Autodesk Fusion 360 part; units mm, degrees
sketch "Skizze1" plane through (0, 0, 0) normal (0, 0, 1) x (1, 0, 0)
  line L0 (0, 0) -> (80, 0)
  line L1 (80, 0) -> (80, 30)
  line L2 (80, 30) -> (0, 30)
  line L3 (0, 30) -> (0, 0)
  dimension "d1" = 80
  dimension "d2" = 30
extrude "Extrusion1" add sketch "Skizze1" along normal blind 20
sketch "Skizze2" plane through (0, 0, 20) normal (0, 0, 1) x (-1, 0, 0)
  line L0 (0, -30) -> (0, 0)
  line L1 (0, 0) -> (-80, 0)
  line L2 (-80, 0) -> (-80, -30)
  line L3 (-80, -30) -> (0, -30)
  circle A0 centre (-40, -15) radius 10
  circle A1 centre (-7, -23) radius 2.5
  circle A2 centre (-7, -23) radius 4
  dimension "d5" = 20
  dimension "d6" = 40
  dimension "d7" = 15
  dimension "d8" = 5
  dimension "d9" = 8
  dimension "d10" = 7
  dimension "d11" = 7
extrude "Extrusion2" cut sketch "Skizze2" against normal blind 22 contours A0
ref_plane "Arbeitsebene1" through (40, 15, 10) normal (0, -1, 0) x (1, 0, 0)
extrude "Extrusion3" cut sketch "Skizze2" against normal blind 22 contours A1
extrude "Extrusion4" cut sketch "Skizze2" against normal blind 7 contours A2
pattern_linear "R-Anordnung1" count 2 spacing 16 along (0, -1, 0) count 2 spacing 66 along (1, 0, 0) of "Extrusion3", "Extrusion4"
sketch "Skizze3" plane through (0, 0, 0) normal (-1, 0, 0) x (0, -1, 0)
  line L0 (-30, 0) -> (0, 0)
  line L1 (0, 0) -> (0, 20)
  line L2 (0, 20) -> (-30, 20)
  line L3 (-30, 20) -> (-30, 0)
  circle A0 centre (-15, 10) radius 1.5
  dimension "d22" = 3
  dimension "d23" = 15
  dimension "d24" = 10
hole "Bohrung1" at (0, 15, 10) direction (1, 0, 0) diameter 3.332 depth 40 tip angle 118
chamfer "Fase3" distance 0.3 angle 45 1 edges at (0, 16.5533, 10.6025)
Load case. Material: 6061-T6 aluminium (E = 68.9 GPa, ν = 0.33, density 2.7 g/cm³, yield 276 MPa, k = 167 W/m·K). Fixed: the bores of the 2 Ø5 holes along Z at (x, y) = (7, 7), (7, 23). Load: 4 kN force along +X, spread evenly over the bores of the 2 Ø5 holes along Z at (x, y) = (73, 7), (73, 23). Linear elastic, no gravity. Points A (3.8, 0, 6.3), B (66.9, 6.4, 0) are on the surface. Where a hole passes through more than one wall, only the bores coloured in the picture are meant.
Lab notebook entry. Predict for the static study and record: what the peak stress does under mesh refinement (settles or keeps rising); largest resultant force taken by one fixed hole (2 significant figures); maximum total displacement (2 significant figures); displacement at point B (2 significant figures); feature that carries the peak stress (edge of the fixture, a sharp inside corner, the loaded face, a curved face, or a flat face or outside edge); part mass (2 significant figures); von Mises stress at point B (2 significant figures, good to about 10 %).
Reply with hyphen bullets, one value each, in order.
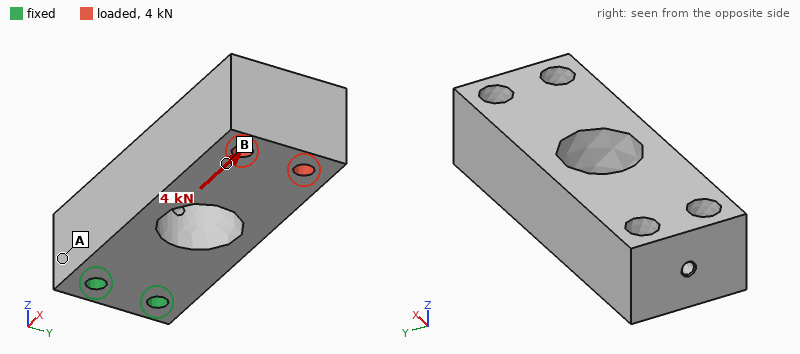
- keeps rising
- 2.0 kN
- 47 µm
- 35 µm
- a sharp inside corner
- 110 g
- 13 MPa
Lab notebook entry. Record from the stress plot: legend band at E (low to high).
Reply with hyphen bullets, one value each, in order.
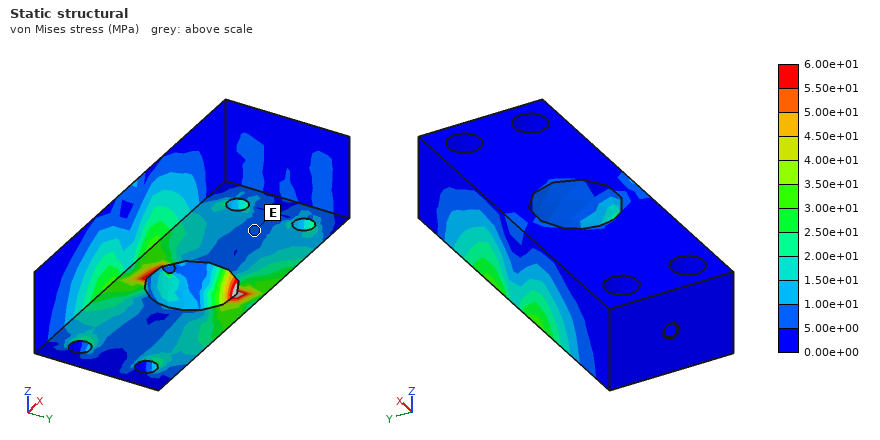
- 5.00e+00 to 1.00e+01 MPa
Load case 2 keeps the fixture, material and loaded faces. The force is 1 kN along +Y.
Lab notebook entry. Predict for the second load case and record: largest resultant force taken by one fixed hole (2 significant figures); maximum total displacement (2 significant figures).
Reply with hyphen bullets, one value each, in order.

- 3.4 kN
- 73 µm
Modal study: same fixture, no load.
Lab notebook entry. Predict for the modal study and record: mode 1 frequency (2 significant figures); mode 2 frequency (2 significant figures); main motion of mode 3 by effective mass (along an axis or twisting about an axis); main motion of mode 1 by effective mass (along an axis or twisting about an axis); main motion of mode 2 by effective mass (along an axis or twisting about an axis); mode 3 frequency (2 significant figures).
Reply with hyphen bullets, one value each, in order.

- 2200 Hz
- 3300 Hz
- twisting about X
- along Z
- along Y
- 7400 Hz
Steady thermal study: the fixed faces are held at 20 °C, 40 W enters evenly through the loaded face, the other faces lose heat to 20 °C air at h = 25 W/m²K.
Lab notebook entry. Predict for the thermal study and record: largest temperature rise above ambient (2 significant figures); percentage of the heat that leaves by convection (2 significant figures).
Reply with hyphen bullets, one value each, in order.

- 39 K
- 12 %
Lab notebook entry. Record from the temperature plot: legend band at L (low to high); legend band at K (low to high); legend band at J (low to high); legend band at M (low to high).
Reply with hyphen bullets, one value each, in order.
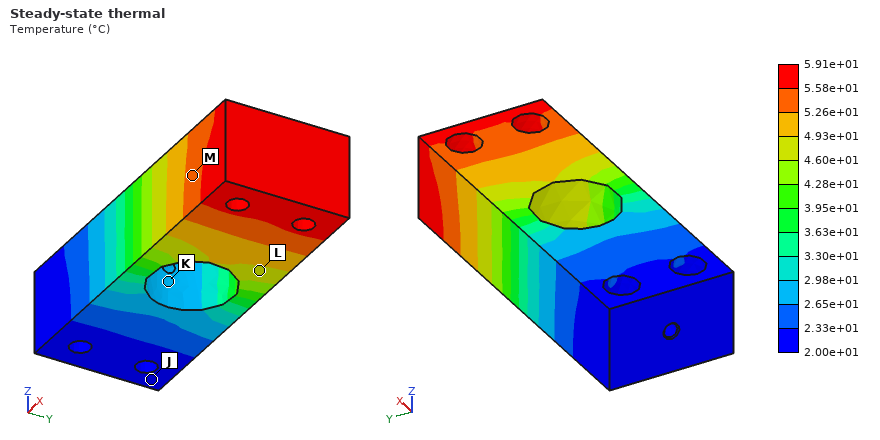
- 4.60e+01 to 4.93e+01 °C
- 2.65e+01 to 2.98e+01 °C
- 2.00e+01 to 2.33e+01 °C
- 5.26e+01 to 5.58e+01 °C
